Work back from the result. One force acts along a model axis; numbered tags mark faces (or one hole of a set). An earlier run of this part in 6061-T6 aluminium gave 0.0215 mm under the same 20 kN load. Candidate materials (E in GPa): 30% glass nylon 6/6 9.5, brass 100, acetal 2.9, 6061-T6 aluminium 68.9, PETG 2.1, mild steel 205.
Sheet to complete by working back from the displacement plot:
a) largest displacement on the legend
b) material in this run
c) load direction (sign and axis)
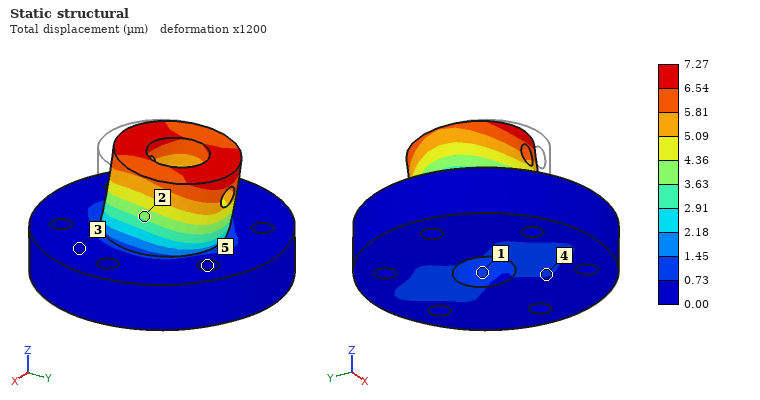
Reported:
7.27 µm
mild steel
+Y
